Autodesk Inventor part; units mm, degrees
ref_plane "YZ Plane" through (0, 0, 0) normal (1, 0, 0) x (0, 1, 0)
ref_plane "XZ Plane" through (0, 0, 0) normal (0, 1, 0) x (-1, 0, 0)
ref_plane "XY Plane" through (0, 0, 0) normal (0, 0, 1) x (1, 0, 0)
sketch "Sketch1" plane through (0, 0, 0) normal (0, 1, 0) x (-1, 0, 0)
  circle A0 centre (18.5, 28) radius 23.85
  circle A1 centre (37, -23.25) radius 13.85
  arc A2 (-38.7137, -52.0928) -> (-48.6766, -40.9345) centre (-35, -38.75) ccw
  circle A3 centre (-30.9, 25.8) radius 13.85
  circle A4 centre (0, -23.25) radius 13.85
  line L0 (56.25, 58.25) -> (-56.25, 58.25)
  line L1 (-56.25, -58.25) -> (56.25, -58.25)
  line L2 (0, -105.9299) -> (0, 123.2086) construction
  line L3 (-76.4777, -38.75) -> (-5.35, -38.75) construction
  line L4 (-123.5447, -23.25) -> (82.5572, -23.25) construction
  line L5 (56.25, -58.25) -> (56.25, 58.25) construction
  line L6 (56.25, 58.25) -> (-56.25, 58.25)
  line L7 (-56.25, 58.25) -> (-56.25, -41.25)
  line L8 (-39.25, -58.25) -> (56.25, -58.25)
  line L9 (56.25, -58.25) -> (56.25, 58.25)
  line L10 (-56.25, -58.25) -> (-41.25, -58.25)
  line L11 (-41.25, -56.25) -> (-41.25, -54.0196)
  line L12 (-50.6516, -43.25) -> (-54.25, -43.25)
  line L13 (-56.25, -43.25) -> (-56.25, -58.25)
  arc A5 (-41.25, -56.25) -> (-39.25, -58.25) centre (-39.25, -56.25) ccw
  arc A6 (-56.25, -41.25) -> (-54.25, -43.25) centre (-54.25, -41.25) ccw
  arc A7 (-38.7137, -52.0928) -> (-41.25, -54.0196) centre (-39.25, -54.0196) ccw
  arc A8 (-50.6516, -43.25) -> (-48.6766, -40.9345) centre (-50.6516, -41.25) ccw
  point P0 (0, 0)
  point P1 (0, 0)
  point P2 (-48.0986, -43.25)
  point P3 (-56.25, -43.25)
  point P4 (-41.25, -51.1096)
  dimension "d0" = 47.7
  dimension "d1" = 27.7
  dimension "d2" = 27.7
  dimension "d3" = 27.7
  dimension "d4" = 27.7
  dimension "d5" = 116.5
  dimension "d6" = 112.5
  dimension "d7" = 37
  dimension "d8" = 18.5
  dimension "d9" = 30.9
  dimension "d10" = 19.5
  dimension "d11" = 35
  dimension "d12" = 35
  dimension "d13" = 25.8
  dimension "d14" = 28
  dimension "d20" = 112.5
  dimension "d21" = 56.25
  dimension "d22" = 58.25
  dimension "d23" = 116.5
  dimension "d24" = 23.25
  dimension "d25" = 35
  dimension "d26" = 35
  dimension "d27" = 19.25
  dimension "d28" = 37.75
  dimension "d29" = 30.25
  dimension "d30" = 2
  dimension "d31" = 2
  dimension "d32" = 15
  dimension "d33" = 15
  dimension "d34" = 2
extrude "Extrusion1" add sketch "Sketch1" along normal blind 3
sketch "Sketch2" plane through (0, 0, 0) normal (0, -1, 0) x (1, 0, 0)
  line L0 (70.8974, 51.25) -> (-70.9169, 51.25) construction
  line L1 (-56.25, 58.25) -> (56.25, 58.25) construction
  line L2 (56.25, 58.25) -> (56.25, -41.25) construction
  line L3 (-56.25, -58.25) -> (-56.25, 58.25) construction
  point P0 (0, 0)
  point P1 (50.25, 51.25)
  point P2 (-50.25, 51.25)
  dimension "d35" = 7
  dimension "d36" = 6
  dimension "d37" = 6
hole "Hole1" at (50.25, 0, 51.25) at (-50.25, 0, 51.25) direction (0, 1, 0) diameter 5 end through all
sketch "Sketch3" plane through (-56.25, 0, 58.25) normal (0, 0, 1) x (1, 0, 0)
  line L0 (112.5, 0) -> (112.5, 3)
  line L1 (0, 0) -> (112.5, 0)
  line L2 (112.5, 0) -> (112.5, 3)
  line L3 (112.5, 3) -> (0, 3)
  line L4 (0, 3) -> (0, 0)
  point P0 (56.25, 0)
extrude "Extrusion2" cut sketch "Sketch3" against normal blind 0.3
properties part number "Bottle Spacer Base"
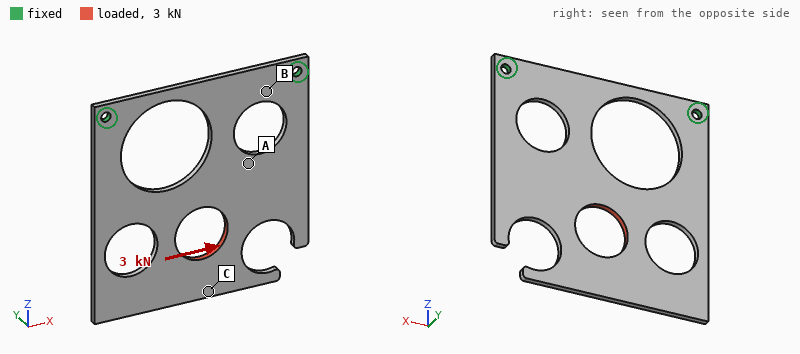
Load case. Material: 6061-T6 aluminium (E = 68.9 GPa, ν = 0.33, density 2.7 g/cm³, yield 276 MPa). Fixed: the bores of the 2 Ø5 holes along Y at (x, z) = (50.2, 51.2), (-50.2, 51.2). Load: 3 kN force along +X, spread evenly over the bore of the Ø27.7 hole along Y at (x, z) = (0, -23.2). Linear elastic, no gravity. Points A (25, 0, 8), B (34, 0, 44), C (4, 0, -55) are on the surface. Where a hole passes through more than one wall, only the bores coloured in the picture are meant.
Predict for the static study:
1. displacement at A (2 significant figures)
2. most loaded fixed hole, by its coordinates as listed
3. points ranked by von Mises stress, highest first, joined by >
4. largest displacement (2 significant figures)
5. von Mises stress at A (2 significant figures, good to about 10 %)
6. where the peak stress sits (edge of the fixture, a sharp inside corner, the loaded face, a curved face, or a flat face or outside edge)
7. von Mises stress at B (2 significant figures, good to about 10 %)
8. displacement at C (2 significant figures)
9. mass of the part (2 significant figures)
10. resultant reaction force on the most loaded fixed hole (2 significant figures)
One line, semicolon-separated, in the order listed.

0.14 mm; (50.2, 51.2); B > A > C; 0.22 mm; 31 MPa; edge of the fixture; 54 MPa; 0.20 mm; 70 g; 2.7 kN
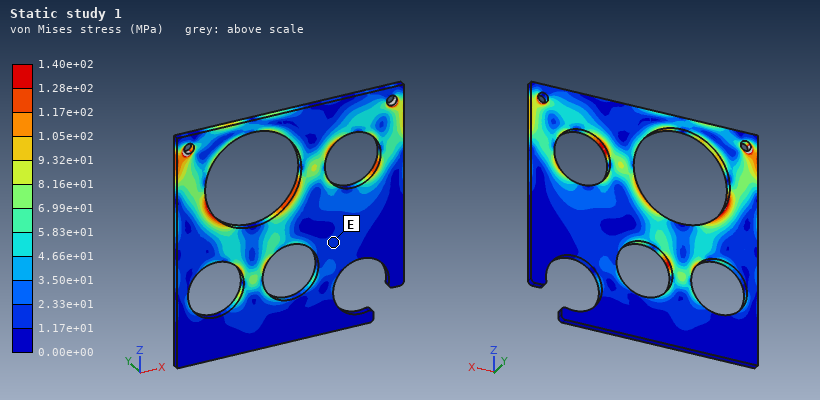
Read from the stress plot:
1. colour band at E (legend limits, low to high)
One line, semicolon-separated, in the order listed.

1.17e+01 to 2.33e+01 MPa
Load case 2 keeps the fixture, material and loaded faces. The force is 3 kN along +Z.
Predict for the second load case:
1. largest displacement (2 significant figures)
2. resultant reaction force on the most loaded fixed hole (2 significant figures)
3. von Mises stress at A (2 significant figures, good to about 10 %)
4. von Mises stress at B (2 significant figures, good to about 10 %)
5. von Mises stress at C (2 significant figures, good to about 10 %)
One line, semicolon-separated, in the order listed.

71 µm; 1.6 kN; 13 MPa; 23 MPa; 8.2 MPa
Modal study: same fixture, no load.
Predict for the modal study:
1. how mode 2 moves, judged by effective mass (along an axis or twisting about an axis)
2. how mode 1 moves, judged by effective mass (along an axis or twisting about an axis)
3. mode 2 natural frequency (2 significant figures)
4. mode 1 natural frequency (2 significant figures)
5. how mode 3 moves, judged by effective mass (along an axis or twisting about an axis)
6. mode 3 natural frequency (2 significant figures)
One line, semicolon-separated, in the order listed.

twisting about Z; along Y; 470 Hz; 150 Hz; along Y; 930 Hz
